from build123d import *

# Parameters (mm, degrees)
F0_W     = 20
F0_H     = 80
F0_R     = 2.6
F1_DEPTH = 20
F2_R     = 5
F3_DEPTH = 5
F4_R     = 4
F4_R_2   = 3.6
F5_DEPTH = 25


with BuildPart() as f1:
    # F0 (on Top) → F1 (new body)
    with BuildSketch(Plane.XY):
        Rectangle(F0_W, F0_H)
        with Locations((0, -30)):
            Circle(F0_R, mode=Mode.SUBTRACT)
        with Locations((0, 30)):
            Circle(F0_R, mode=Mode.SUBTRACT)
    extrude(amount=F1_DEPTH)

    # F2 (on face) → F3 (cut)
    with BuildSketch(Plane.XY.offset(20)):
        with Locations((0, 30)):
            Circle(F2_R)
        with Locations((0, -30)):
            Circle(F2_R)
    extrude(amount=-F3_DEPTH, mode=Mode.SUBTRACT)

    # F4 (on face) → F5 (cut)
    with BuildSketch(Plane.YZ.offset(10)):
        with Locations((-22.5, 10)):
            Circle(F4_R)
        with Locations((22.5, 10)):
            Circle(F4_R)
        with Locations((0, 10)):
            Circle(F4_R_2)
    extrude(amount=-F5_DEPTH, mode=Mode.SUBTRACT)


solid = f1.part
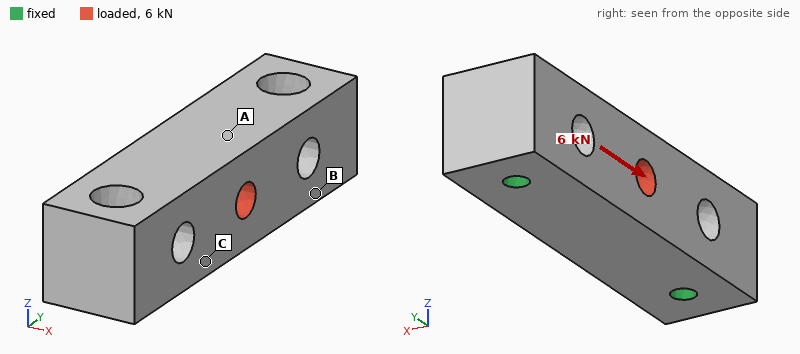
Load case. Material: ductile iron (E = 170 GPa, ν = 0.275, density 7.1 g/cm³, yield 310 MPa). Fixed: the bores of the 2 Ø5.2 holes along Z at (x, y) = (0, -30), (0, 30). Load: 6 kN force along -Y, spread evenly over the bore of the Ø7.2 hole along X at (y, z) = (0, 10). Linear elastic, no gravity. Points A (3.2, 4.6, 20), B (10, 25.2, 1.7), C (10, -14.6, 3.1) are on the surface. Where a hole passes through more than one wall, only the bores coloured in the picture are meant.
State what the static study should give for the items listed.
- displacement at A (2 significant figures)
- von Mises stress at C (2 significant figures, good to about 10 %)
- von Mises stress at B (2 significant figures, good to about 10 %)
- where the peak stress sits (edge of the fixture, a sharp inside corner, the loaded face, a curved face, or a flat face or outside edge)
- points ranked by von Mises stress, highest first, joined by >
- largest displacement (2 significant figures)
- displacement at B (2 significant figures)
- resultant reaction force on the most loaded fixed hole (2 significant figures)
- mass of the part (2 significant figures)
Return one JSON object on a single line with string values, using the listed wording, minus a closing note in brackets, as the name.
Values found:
{"displacement at A": "1.8 µm", "von Mises stress at C": "11 MPa", "von Mises stress at B": "7.5 MPa", "where the peak stress sits": "a curved face", "points ranked by von Mises stress, highest first, joined by >": "C > B > A", "largest displacement": "2.4 µm", "displacement at B": "0.80 µm", "resultant reaction force on the most loaded fixed hole": "3.0 kN", "mass of the part": "200 g"}
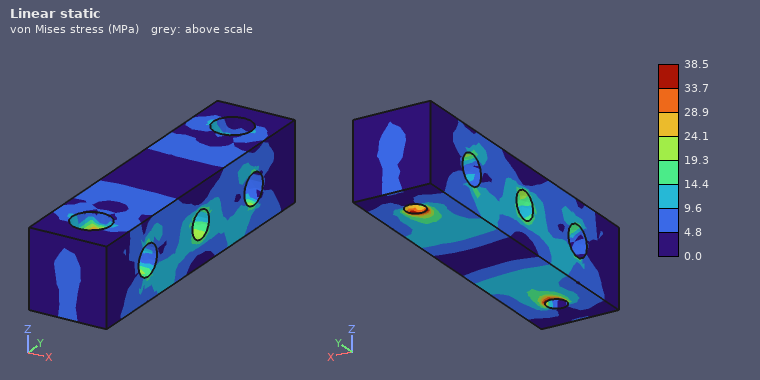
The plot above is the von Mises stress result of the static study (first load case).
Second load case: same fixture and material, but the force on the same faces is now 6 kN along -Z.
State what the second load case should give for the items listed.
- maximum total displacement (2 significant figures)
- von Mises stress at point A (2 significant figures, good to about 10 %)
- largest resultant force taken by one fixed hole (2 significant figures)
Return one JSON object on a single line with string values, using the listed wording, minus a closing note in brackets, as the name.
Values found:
{"maximum total displacement": "12 µm", "von Mises stress at point A": "39 MPa", "largest resultant force taken by one fixed hole": "3.2 kN"}
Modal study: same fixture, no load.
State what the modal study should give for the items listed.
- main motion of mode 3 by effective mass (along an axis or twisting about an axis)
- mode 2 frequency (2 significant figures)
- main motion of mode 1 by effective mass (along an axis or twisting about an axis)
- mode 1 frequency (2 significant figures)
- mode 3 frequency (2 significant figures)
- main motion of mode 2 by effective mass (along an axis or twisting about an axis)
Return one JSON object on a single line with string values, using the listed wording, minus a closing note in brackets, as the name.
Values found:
{"main motion of mode 3 by effective mass": "twisting about Y", "mode 2 frequency": "13 kHz", "main motion of mode 1 by effective mass": "along X", "mode 1 frequency": "12 kHz", "mode 3 frequency": "18 kHz", "main motion of mode 2 by effective mass": "along Z"}
